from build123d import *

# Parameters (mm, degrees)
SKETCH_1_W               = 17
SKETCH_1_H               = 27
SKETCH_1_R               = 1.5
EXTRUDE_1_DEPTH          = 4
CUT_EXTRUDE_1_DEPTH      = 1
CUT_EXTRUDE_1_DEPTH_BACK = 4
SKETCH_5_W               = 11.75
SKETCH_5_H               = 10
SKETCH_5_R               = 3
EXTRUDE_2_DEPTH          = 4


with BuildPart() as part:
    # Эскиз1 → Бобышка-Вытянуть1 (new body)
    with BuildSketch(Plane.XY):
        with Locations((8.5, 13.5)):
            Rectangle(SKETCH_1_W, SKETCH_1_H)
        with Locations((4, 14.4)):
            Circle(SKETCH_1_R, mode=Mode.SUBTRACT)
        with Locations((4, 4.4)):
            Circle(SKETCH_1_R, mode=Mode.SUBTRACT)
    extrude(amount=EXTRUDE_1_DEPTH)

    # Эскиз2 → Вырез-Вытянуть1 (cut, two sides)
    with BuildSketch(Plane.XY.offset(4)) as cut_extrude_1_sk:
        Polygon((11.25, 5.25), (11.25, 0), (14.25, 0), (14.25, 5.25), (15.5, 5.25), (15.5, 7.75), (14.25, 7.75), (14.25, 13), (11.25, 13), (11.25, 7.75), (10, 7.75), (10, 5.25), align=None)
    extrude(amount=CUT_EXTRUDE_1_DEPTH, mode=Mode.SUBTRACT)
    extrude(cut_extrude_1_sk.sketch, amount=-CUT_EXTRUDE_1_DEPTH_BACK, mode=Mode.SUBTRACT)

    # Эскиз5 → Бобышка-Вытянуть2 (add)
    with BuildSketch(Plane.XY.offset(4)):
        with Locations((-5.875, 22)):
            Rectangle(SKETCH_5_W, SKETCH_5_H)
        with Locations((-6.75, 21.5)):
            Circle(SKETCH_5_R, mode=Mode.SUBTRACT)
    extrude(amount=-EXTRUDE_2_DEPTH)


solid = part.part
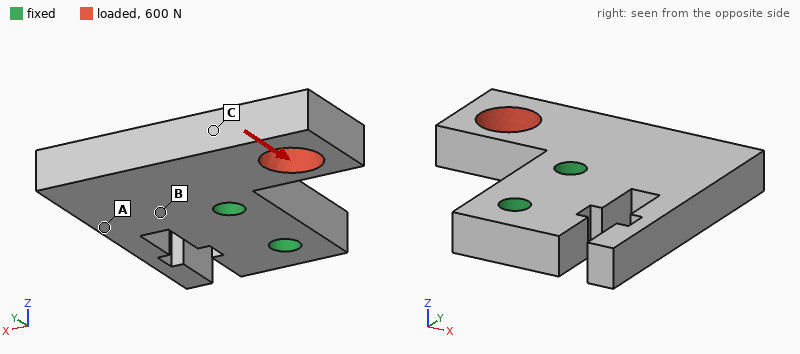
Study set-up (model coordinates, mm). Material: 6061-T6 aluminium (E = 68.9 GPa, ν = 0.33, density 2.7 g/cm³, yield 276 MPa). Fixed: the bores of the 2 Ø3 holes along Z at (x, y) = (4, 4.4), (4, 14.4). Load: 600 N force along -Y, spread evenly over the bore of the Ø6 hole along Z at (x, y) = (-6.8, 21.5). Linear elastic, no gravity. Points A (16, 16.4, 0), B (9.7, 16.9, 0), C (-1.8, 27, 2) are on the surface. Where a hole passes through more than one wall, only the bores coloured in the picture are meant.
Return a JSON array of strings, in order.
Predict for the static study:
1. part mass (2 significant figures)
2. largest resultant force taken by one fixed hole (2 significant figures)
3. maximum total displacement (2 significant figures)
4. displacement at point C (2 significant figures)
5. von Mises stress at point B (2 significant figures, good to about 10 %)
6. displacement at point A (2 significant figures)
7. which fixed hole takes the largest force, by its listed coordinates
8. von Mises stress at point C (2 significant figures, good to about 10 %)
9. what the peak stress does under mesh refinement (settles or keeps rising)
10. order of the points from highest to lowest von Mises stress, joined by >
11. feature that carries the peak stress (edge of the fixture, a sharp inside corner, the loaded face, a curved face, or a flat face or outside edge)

["5.3 g", "890 N", "74 µm", "33 µm", "33 MPa", "15 µm", "(4, 14.4)", "70 MPa", "keeps rising", "C > B > A", "a sharp inside corner"]
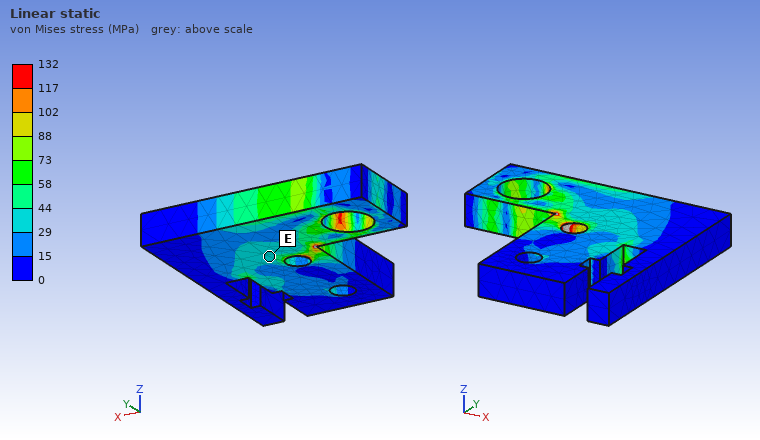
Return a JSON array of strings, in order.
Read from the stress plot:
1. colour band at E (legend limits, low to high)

["29 to 44 MPa"]
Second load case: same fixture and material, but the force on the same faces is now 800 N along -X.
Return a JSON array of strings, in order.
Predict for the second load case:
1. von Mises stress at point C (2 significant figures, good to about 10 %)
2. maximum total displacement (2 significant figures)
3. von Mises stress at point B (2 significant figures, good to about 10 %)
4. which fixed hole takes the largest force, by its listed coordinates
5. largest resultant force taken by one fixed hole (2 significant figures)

["26 MPa", "28 µm", "27 MPa", "(4, 14.4)", "1.1 kN"]
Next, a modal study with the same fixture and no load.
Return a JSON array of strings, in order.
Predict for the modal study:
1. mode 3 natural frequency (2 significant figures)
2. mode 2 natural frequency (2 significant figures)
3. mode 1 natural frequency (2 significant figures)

["10 kHz", "9400 Hz", "8600 Hz"]
